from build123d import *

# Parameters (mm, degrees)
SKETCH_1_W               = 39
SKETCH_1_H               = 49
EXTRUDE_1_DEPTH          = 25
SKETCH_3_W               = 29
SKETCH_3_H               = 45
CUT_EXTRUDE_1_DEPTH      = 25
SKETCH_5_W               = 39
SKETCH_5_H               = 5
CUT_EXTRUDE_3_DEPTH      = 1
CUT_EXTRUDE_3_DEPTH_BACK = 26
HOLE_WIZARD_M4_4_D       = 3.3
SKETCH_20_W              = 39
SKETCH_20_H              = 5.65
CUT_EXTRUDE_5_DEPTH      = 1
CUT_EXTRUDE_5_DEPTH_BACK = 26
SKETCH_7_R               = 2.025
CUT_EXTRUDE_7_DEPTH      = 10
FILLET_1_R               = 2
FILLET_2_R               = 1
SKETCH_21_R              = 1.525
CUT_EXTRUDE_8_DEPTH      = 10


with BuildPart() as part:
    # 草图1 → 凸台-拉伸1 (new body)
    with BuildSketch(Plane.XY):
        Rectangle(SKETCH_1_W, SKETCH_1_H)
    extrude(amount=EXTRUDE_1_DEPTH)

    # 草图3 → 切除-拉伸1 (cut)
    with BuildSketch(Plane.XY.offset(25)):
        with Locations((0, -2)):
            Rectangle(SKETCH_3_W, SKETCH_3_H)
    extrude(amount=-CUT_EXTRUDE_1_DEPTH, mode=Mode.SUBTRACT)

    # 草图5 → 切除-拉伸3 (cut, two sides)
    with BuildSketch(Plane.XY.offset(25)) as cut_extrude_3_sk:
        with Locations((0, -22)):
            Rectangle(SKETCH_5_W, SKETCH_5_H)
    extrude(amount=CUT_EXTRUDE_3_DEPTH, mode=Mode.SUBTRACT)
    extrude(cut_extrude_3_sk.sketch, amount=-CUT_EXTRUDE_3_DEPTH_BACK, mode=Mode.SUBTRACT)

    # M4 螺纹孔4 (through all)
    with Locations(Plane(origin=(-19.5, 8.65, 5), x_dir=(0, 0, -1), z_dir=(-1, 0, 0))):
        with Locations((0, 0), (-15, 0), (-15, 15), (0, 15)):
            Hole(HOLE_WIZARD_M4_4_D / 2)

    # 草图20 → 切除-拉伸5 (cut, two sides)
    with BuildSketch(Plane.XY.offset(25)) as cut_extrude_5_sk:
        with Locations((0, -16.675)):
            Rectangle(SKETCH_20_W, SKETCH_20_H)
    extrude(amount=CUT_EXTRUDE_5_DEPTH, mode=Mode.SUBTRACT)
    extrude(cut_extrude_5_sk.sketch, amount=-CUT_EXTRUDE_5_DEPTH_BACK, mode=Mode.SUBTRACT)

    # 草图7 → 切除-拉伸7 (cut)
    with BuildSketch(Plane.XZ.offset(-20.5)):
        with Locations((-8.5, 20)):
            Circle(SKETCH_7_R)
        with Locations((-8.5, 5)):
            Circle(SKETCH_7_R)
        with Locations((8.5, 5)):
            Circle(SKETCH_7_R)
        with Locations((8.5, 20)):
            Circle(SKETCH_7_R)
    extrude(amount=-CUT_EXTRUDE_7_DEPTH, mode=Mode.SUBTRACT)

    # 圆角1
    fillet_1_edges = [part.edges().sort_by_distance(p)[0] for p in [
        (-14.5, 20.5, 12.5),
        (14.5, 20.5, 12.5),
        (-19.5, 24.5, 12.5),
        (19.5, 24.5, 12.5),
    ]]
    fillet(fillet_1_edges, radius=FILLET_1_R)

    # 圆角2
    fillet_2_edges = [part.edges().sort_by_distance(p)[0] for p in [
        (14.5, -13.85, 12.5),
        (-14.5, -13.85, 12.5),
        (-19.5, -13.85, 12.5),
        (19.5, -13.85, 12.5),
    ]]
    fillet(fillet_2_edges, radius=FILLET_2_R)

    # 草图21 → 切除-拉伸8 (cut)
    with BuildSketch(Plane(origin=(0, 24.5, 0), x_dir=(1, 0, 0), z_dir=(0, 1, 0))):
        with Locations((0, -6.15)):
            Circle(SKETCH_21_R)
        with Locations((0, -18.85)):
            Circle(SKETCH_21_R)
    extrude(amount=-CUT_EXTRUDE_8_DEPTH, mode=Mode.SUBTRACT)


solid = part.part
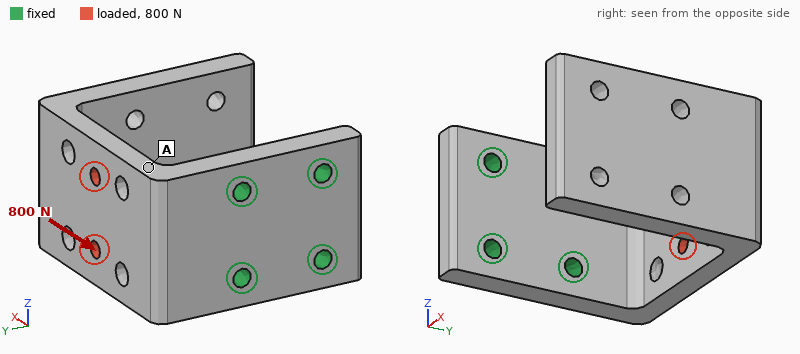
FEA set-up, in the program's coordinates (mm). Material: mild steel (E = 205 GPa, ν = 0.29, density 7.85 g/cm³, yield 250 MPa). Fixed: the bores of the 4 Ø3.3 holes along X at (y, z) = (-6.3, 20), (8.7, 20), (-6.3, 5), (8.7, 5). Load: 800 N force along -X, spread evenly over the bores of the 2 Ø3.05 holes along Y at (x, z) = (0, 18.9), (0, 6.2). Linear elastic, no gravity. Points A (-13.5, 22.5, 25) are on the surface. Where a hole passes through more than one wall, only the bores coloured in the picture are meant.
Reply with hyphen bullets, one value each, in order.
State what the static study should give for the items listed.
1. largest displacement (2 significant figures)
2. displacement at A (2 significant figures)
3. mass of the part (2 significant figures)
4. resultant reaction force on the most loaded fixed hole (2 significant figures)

- 63 µm
- 15 µm
- 93 g
- 470 N
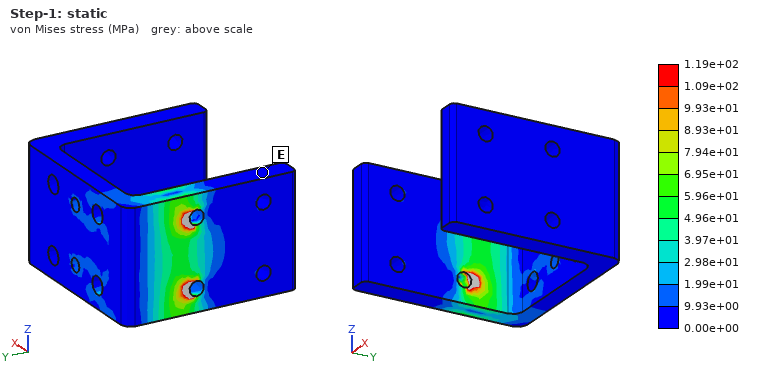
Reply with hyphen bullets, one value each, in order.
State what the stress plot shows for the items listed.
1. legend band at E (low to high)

- 0.00e+00 to 9.93e+00 MPa
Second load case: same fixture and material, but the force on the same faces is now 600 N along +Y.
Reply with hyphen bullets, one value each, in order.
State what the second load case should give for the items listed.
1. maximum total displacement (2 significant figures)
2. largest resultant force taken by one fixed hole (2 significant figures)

- 0.24 mm
- 290 N
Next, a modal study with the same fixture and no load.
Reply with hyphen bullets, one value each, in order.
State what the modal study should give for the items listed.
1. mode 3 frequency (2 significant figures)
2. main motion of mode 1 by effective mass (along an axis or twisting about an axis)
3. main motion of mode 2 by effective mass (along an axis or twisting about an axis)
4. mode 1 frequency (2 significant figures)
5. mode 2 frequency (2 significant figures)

- 2100 Hz
- along Y
- along Z
- 730 Hz
- 1200 Hz
